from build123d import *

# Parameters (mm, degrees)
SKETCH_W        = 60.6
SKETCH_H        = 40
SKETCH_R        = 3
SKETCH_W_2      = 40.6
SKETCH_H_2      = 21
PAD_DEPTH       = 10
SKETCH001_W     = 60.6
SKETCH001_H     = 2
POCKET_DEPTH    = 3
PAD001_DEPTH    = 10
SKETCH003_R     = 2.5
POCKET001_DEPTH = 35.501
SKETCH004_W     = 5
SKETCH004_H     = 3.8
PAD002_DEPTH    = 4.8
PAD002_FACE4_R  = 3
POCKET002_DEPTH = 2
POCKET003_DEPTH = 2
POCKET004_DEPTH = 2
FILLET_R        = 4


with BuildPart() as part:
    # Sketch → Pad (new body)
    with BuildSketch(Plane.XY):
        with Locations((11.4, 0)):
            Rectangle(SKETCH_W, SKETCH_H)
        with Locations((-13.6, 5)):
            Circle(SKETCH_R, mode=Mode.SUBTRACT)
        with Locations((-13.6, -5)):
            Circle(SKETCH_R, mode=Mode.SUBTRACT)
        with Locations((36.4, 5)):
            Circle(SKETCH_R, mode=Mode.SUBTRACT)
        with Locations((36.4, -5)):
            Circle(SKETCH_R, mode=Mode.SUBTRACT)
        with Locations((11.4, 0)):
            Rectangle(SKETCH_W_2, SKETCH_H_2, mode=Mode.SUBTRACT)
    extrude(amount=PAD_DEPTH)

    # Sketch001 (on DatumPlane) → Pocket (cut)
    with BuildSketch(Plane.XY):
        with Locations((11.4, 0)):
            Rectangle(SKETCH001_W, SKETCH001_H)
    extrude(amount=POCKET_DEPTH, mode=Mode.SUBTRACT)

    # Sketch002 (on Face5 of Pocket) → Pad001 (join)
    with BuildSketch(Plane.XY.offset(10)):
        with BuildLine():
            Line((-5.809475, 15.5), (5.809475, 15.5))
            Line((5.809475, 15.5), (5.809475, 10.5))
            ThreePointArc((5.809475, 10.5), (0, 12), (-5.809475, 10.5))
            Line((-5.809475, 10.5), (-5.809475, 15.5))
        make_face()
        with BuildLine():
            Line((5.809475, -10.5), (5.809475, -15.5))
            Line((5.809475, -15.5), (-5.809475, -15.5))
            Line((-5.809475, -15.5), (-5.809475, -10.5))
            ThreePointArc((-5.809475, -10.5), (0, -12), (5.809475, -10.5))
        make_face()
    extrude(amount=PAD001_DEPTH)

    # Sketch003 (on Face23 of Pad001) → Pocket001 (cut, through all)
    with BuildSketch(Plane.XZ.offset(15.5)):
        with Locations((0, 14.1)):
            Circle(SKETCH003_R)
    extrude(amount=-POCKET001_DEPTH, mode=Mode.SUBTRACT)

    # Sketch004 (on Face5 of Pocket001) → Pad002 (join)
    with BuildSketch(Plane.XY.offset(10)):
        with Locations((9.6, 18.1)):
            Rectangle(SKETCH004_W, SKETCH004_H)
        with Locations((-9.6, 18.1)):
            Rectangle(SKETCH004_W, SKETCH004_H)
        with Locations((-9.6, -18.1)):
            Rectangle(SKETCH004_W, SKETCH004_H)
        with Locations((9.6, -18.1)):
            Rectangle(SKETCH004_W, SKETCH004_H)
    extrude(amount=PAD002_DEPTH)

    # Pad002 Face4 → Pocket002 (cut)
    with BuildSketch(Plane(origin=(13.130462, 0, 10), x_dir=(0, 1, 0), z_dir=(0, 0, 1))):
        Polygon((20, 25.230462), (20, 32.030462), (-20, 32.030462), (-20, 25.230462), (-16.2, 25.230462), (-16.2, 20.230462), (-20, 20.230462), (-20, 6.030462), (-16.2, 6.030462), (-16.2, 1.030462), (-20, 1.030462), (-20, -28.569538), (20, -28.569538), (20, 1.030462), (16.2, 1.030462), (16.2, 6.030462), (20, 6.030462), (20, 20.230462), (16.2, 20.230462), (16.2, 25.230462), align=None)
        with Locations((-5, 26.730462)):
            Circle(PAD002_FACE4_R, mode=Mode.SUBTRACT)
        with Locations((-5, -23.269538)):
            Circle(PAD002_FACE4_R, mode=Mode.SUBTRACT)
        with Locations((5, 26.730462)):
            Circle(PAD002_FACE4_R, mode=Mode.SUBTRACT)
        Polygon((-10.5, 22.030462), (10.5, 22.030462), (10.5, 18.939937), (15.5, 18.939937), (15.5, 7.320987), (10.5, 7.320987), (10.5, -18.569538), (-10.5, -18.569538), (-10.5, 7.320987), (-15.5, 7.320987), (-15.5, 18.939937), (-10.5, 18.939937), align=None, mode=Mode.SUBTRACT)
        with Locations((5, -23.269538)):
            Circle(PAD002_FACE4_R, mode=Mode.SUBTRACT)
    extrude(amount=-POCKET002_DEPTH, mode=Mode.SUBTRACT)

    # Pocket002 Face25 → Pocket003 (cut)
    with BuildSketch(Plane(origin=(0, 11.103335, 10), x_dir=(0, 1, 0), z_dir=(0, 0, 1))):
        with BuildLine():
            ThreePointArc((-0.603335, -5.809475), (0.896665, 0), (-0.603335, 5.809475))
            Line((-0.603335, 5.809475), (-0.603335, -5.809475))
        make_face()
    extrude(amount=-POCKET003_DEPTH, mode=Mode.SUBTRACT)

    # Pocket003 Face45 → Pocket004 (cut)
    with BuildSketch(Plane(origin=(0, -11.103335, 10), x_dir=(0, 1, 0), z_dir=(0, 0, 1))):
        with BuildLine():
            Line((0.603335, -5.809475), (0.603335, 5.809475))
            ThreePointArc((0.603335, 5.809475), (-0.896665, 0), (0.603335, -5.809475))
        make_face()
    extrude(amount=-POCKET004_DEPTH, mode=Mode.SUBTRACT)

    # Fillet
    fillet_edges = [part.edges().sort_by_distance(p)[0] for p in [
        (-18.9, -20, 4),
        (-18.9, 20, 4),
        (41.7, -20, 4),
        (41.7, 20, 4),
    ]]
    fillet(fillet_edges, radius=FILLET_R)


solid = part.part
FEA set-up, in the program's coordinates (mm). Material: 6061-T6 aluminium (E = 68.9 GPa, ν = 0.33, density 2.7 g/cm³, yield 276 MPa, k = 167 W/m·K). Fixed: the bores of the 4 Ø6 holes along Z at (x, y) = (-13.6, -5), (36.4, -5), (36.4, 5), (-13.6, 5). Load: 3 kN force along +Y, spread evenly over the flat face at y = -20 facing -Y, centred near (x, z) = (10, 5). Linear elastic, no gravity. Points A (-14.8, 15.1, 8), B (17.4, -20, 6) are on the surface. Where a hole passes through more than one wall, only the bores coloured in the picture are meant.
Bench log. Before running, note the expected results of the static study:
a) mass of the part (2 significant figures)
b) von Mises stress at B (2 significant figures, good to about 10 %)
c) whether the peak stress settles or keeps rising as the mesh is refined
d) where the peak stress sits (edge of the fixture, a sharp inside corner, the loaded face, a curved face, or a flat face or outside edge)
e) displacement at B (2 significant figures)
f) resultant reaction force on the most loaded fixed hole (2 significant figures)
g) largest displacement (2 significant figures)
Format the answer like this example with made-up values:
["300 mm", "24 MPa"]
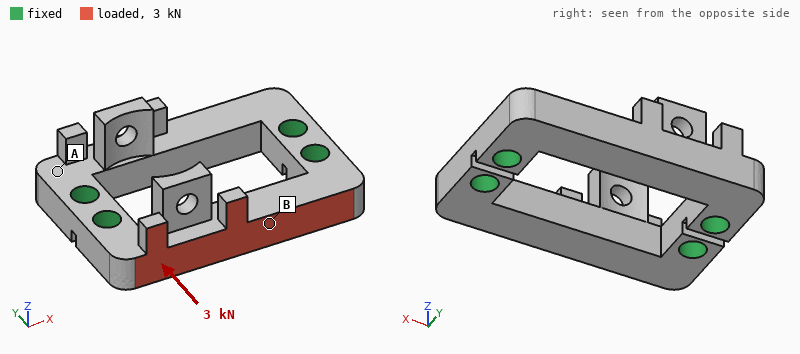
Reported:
["35 g", "55 MPa", "keeps rising", "a sharp inside corner", "34 µm", "1.9 kN", "65 µm"]
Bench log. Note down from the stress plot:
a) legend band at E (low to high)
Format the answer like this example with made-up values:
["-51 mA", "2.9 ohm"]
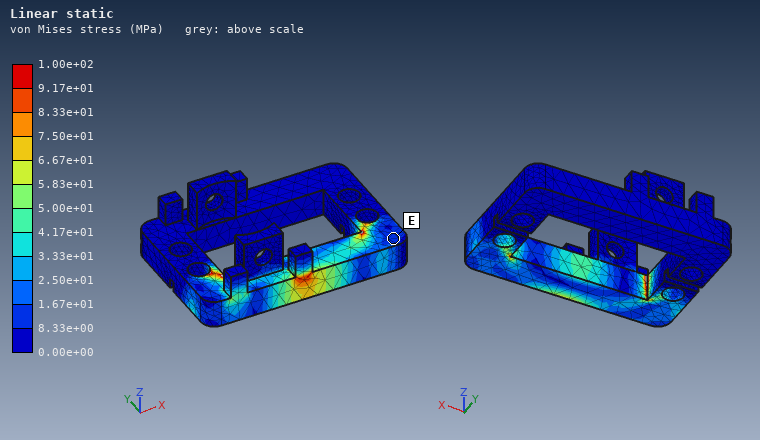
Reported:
["8.33e+00 to 1.67e+01 MPa"]
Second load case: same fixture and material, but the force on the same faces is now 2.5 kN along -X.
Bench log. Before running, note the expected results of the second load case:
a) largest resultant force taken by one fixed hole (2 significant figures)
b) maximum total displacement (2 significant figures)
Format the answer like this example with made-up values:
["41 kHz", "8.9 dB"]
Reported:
["1.4 kN", "24 µm"]
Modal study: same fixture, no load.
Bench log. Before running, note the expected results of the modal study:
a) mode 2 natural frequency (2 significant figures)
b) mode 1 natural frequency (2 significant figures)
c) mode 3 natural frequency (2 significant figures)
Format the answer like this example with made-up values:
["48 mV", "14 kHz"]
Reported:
["9500 Hz", "9500 Hz", "12 kHz"]
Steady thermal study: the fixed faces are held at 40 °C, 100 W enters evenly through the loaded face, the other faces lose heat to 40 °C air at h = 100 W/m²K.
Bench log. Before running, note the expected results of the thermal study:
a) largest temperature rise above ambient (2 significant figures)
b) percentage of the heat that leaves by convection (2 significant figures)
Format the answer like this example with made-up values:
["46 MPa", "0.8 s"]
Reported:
["70 K", "9.3 %"]
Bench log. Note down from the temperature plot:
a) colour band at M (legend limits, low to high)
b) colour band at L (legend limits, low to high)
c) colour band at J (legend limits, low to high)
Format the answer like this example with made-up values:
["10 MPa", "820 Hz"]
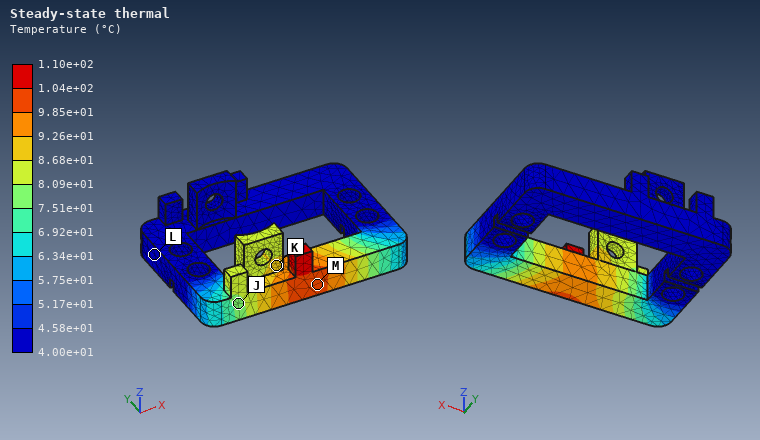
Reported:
["9.85e+01 to 1.04e+02 °C", "4.00e+01 to 4.58e+01 °C", "7.51e+01 to 8.09e+01 °C"]
